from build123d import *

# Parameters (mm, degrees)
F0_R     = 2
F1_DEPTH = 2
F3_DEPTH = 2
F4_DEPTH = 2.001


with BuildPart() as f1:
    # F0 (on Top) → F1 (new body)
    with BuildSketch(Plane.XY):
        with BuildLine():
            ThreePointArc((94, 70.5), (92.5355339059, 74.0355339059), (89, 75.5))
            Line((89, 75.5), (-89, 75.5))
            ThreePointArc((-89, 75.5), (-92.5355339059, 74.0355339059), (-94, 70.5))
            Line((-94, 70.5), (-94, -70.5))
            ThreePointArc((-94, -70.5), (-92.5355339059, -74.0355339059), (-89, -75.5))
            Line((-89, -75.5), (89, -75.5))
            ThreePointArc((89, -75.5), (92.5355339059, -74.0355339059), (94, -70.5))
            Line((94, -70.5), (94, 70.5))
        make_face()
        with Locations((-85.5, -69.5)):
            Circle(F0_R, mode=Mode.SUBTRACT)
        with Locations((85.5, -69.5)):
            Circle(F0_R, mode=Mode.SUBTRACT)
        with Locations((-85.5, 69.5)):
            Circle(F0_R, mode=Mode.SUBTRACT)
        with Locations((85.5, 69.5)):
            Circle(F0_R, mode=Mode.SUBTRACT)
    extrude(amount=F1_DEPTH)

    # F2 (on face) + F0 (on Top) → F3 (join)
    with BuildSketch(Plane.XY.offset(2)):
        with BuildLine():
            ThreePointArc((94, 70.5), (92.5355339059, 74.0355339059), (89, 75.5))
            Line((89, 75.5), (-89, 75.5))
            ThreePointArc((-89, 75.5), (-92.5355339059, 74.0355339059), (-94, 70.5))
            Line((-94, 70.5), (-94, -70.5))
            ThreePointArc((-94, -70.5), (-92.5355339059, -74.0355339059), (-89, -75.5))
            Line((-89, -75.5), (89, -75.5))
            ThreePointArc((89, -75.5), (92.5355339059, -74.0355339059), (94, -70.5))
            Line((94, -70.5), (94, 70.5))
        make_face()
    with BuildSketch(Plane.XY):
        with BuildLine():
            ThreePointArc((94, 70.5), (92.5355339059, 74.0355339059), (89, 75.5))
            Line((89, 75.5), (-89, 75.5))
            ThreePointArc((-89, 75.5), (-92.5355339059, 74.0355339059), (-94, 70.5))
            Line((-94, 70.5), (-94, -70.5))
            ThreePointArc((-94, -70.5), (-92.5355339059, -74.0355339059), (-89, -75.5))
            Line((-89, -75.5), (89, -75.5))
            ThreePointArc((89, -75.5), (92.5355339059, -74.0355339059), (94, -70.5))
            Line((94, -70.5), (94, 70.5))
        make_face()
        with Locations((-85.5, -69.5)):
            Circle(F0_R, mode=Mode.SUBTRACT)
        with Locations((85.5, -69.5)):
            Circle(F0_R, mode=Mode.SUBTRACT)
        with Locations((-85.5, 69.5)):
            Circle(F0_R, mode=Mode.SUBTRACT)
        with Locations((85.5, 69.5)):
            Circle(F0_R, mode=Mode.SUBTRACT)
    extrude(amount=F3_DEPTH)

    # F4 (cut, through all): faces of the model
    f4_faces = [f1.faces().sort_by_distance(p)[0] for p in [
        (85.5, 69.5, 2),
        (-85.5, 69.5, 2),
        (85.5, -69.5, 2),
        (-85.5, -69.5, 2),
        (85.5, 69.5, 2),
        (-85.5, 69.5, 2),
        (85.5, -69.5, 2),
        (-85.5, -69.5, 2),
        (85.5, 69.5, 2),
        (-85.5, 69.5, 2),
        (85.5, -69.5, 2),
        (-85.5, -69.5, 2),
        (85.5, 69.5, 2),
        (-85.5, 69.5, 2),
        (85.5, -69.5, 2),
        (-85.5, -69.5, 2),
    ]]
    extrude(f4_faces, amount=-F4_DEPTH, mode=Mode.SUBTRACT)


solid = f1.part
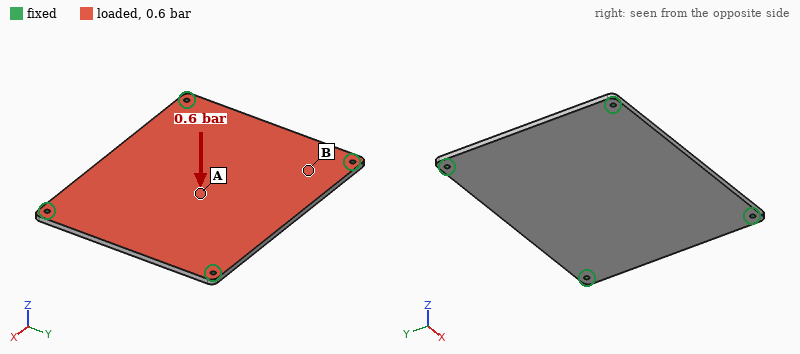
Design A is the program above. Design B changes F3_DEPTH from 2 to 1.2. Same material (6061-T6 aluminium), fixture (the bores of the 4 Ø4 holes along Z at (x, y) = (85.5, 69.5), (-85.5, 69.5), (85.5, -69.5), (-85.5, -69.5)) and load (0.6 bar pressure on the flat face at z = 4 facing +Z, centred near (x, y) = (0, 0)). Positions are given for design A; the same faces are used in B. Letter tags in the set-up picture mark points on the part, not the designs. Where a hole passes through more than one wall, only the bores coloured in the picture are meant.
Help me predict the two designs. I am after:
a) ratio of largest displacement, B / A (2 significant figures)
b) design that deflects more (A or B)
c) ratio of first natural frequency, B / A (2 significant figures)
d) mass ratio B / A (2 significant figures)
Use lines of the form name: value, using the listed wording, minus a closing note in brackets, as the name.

ratio of largest displacement, B / A: 1.9
design that deflects more: B
ratio of first natural frequency, B / A: 0.81
mass ratio B / A: 0.80
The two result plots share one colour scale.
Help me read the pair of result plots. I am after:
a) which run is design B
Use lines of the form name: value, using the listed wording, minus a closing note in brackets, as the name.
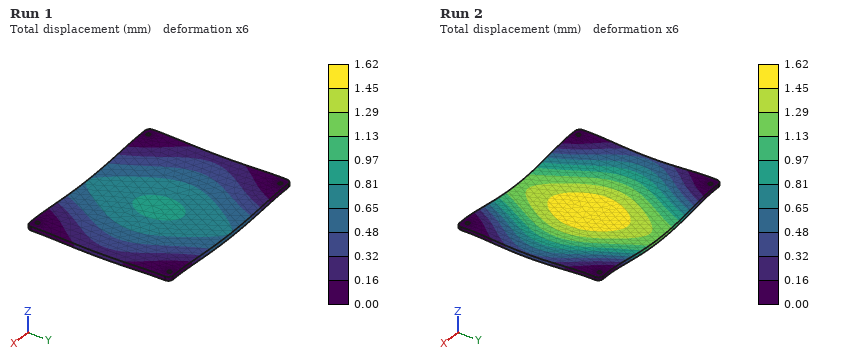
which run is design B: Run 2
